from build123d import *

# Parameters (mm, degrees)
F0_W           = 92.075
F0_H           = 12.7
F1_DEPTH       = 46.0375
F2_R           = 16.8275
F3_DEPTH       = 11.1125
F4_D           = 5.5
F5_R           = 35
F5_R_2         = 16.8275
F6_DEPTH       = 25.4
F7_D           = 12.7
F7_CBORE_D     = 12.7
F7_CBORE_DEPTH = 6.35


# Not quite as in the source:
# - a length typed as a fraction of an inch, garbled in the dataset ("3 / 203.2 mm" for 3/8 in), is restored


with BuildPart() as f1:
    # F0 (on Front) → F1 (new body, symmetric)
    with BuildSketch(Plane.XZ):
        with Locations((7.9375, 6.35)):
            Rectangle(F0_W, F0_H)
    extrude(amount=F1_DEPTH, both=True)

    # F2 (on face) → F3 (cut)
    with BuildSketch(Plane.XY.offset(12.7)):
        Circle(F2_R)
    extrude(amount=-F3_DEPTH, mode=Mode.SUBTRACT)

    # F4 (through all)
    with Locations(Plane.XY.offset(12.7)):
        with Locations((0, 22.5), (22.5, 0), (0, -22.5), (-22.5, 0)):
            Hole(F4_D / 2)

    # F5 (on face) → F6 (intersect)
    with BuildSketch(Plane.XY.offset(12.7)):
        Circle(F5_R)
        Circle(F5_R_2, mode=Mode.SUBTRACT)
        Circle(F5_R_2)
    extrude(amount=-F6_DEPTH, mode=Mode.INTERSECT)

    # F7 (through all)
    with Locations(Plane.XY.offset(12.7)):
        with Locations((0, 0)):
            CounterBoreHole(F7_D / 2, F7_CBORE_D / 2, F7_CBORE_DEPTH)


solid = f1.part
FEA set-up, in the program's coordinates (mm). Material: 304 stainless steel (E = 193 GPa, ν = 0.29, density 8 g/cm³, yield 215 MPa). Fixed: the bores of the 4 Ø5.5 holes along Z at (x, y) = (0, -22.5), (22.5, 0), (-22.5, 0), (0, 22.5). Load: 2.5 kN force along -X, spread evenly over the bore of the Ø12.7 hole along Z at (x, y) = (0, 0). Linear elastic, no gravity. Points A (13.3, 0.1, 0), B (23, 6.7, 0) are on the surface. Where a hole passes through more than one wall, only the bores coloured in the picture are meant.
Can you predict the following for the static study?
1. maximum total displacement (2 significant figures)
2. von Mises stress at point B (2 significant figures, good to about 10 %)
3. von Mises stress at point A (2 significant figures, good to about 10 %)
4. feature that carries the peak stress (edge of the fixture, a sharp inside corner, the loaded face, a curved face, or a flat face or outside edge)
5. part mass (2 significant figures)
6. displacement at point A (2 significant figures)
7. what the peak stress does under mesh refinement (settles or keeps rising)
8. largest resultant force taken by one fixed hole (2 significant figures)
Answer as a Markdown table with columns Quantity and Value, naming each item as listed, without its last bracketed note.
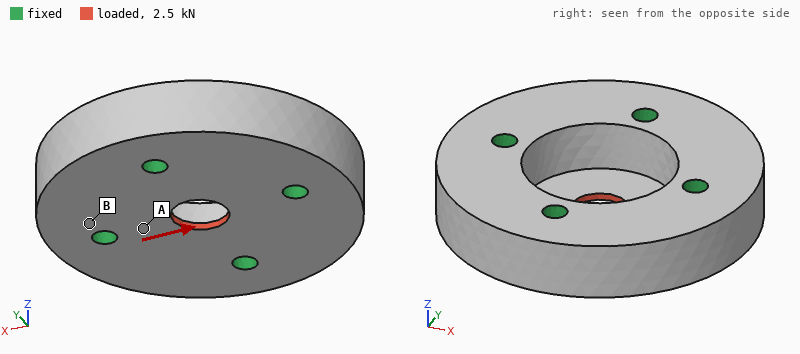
| Quantity | Value |
|---|---|
| maximum total displacement | 2.7 µm |
| von Mises stress at point B | 6.5 MPa |
| von Mises stress at point A | 32 MPa |
| feature that carries the peak stress | a sharp inside corner |
| part mass | 300 g |
| displacement at point A | 1.3 µm |
| what the peak stress does under mesh refinement | keeps rising |
| largest resultant force taken by one fixed hole | 730 N |
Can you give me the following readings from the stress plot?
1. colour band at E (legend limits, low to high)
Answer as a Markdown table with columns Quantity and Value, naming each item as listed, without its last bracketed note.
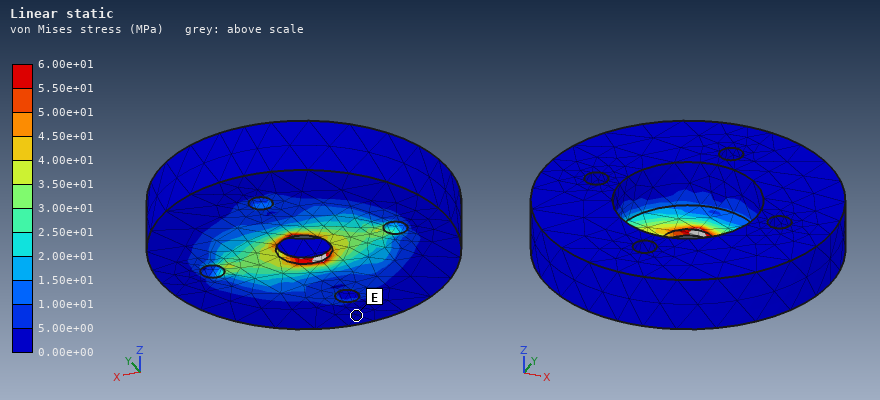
| Quantity | Value |
|---|---|
| colour band at E | 0.00e+00 to 5.00e+00 MPa |
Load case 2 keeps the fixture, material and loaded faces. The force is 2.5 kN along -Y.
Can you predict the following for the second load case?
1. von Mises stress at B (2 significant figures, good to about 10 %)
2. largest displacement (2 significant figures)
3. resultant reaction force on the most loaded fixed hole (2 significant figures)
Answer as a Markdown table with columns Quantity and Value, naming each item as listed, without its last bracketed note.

| Quantity | Value |
|---|---|
| von Mises stress at B | 4.9 MPa |
| largest displacement | 2.7 µm |
| resultant reaction force on the most loaded fixed hole | 730 N |
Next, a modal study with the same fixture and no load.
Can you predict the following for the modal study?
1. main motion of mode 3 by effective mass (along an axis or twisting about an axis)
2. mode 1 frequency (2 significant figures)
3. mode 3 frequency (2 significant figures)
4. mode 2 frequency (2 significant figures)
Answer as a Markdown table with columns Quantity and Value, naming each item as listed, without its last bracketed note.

| Quantity | Value |
|---|---|
| main motion of mode 3 by effective mass | twisting about Y |
| mode 1 frequency | 15 kHz |
| mode 3 frequency | 21 kHz |
| mode 2 frequency | 20 kHz |
